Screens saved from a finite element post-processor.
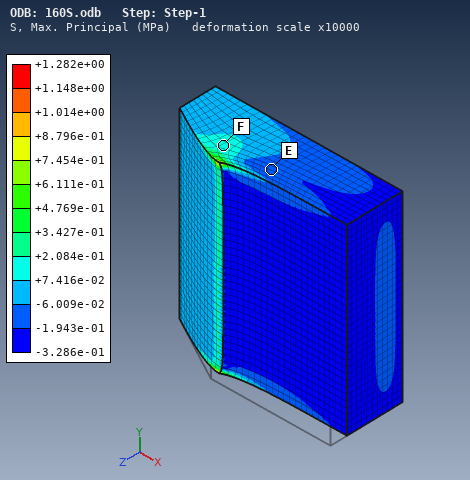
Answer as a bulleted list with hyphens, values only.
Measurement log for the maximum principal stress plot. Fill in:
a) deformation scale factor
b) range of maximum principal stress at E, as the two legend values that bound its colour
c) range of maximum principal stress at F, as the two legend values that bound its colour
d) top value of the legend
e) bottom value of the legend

- 10000
- -1.943e-01 to -6.009e-02 MPa
- +7.416e-02 to +2.084e-01 MPa
- +1.282e+00 MPa
- -3.286e-01 MPa
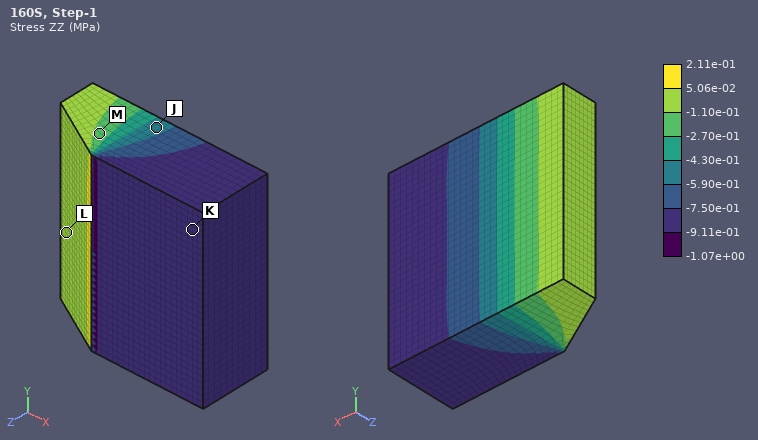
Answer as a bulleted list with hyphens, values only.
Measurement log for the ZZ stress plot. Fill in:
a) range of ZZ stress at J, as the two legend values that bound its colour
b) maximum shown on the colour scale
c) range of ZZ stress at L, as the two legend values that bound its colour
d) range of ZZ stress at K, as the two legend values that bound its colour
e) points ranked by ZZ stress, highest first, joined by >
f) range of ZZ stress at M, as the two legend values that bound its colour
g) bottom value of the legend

- -5.90e-01 to -4.30e-01 MPa
- 2.11e-01 MPa
- -1.10e-01 to 5.06e-02 MPa
- -9.11e-01 to -7.50e-01 MPa
- L > M > J > K
- -2.70e-01 to -1.10e-01 MPa
- -1.07e+00 MPa
